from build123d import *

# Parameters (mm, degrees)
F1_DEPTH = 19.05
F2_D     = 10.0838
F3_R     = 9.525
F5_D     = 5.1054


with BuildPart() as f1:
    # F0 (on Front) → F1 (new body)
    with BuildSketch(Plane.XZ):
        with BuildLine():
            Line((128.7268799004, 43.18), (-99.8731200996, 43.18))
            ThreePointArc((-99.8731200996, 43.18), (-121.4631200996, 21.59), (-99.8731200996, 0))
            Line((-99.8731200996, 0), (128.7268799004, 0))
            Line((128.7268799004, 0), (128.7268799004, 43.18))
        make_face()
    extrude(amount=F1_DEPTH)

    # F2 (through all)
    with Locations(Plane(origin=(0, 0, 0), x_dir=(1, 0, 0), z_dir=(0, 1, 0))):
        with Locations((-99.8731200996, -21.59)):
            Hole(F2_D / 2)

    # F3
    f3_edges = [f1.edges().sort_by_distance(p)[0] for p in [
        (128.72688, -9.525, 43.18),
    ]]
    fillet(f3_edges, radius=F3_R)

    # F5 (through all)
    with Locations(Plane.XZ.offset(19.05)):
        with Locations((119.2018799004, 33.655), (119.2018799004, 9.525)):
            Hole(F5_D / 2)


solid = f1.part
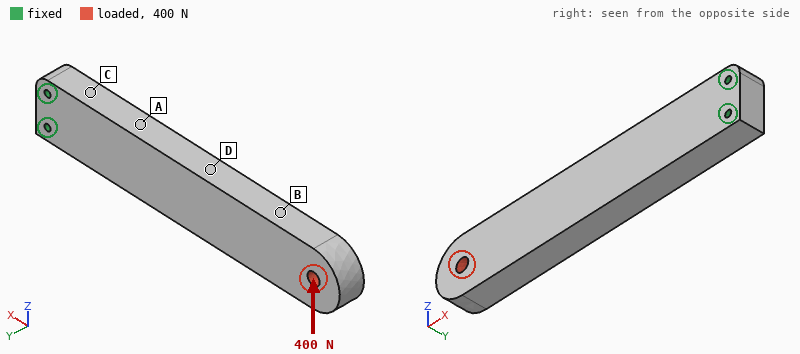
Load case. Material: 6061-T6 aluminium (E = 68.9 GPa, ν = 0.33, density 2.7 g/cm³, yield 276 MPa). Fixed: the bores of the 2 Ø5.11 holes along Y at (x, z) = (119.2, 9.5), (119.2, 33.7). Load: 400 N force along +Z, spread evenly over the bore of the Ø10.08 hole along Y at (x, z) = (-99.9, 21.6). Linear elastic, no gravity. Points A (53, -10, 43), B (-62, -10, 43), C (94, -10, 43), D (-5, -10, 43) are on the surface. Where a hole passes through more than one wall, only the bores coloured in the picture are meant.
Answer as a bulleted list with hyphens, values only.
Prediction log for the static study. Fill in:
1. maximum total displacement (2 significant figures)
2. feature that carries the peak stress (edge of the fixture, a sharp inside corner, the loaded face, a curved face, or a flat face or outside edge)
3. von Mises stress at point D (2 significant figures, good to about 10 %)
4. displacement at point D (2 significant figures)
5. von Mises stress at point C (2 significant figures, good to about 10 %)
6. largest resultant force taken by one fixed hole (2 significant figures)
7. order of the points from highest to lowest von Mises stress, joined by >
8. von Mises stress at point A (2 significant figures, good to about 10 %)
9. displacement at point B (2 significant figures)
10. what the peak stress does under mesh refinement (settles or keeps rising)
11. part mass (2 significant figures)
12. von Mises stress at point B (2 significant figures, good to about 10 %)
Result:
- 0.20 mm
- edge of the fixture
- 6.4 MPa
- 0.073 mm
- 13 MPa
- 3.3 kN
- C > A > D > B
- 10 MPa
- 0.13 mm
- keeps rising
- 540 g
- 2.5 MPa
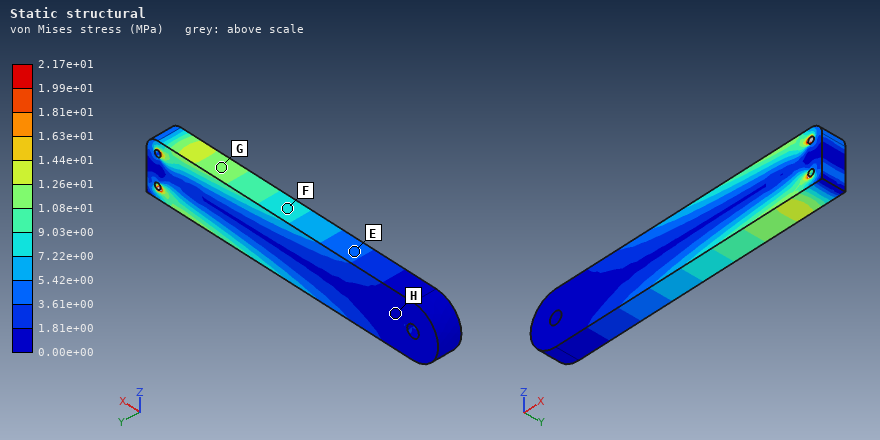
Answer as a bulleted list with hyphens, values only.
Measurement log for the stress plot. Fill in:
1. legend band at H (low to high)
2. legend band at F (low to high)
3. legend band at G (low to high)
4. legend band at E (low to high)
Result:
- 0.00e+00 to 1.81e+00 MPa
- 7.22e+00 to 9.03e+00 MPa
- 1.08e+01 to 1.26e+01 MPa
- 3.61e+00 to 5.42e+00 MPa
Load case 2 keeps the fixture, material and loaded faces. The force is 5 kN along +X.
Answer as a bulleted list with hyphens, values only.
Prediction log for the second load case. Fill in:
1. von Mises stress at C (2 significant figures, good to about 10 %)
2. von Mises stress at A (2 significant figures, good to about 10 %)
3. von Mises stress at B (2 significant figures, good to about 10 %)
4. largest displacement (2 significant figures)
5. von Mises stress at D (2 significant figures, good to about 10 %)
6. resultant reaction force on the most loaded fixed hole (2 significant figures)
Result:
- 5.9 MPa
- 6.1 MPa
- 6.1 MPa
- 22 µm
- 6.1 MPa
- 2.5 kN
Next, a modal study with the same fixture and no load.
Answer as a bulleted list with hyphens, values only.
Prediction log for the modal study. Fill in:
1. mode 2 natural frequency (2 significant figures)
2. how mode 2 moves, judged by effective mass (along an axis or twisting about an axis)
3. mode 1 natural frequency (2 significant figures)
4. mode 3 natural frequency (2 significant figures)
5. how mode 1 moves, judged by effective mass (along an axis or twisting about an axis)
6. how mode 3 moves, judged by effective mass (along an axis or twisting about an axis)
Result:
- 600 Hz
- along Z
- 280 Hz
- 1700 Hz
- along Y
- along Y
